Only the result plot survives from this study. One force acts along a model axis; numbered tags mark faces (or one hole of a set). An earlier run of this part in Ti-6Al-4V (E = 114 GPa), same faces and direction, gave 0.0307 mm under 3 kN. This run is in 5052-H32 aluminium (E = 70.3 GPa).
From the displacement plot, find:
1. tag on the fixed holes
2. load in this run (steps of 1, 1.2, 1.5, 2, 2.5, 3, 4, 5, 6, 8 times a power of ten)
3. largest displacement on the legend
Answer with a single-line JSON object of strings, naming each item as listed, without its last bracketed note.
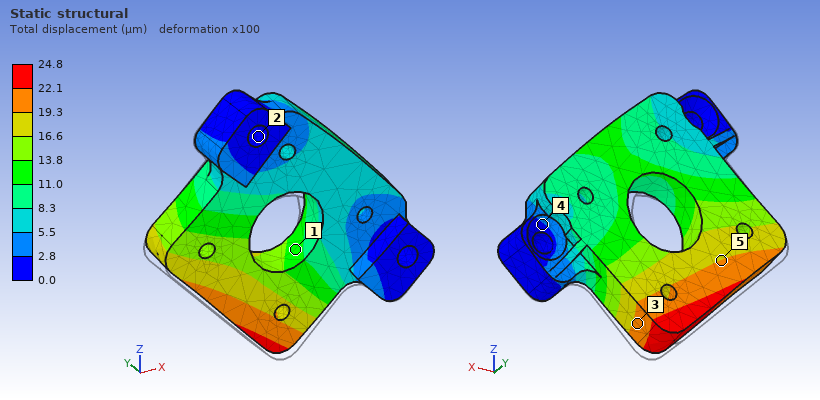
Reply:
{"tag on the fixed holes": "2", "load in this run": "1.5 kN", "largest displacement on the legend": "24.8 µm"}
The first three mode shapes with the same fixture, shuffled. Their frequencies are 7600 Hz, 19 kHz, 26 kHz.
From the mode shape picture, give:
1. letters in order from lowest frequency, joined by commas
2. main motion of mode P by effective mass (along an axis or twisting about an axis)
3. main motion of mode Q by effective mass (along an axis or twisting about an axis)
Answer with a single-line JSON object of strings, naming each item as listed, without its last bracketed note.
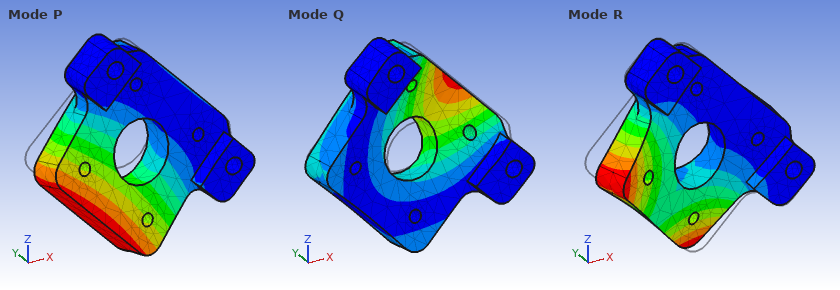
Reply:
{"letters in order from lowest frequency, joined by commas": "P, R, Q", "main motion of mode P by effective mass": "along Y", "main motion of mode Q by effective mass": "along Y"}
